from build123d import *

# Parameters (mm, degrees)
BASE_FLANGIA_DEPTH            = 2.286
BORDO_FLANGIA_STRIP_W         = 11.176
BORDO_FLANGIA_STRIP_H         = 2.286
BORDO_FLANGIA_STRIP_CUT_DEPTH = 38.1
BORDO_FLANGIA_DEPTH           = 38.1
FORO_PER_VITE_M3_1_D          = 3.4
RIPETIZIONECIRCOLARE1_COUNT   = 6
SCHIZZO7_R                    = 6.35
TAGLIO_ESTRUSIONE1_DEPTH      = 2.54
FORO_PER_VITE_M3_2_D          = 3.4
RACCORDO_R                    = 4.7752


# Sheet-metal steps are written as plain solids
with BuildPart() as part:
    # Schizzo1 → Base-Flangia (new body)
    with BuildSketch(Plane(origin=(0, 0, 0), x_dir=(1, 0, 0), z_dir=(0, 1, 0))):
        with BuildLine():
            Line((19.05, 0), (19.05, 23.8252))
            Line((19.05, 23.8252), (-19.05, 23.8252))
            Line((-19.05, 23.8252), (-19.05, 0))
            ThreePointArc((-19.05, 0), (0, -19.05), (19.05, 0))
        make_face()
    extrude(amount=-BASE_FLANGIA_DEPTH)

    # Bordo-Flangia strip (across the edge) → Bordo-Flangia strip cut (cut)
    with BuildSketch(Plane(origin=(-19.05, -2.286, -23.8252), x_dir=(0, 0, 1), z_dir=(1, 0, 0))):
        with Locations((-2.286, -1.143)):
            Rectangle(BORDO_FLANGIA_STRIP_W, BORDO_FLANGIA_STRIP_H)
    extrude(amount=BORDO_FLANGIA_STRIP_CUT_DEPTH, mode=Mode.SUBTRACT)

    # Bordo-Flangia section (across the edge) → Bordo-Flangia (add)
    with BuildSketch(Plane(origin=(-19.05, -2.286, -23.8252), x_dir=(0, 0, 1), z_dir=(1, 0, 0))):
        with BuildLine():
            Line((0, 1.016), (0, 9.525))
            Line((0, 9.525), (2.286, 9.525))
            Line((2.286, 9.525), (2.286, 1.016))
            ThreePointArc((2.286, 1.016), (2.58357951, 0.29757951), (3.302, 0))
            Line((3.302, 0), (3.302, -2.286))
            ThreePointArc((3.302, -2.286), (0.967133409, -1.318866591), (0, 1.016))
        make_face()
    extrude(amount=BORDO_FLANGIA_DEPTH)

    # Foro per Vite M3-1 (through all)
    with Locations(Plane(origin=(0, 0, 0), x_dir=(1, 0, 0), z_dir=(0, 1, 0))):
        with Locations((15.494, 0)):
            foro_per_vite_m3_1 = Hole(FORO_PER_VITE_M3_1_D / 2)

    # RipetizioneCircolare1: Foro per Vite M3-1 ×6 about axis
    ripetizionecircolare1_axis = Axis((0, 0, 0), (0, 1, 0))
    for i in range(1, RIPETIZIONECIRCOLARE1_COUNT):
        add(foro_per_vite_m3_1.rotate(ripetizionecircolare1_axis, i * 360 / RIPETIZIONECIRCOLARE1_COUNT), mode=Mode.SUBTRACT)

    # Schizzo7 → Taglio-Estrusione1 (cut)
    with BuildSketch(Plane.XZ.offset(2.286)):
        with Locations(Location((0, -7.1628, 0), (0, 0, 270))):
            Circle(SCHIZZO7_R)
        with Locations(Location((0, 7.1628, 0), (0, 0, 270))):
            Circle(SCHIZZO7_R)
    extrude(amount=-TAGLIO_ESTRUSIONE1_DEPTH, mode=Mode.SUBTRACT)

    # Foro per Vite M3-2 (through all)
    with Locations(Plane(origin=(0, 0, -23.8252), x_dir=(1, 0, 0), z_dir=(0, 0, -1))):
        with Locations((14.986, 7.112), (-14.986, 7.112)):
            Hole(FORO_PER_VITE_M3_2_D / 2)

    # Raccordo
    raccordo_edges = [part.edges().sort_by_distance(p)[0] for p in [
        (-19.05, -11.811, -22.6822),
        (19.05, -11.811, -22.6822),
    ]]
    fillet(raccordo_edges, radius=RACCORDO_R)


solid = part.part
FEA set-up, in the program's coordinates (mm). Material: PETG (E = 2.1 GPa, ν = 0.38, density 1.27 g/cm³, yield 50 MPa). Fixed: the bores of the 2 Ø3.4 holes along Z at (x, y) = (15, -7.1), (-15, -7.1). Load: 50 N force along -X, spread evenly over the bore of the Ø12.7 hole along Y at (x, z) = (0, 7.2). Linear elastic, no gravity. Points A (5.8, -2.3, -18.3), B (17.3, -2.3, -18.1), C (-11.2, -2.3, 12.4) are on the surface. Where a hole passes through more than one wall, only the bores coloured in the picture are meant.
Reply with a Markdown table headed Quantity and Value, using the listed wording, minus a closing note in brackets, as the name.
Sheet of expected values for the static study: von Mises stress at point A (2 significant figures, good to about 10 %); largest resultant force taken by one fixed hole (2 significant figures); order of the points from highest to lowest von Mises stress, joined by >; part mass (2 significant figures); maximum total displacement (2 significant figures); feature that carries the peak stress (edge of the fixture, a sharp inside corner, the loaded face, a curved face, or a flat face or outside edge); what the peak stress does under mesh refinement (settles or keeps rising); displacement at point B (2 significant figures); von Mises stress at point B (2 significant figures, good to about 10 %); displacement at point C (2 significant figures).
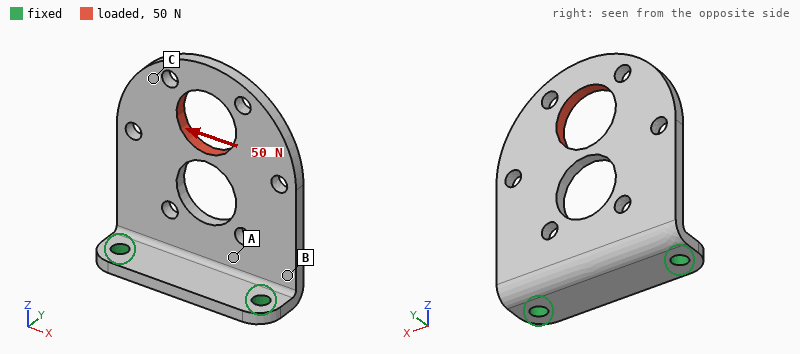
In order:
| Quantity | Value |
|---|---|
| von Mises stress at point A | 4.0 MPa |
| largest resultant force taken by one fixed hole | 56 N |
| order of the points from highest to lowest von Mises stress, joined by > | B > A > C |
| part mass | 4.3 g |
| maximum total displacement | 0.40 mm |
| feature that carries the peak stress | edge of the fixture |
| what the peak stress does under mesh refinement | keeps rising |
| displacement at point B | 0.13 mm |
| von Mises stress at point B | 7.0 MPa |
| displacement at point C | 0.38 mm |
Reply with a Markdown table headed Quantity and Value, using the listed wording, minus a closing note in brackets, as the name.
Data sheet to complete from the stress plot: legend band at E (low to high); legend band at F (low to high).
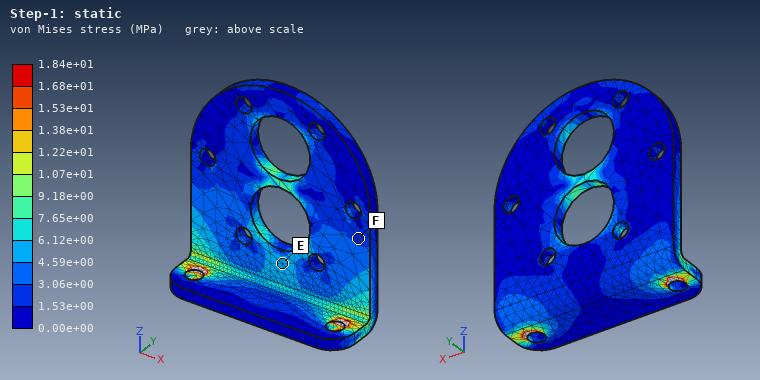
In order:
| Quantity | Value |
|---|---|
| legend band at E | 4.59e+00 to 6.12e+00 MPa |
| legend band at F | 1.53e+00 to 3.06e+00 MPa |
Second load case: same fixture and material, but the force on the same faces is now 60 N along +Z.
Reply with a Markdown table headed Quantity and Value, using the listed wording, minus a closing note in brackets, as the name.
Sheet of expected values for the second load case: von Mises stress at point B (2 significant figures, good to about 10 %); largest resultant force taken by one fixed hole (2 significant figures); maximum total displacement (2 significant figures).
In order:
| Quantity | Value |
|---|---|
| von Mises stress at point B | 2.2 MPa |
| largest resultant force taken by one fixed hole | 30 N |
| maximum total displacement | 0.61 mm |
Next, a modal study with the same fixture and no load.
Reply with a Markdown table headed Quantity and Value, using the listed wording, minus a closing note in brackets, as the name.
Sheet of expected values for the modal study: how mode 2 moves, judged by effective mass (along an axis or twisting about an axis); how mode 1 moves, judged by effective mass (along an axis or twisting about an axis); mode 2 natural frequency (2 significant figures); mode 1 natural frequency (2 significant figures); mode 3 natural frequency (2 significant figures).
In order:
| Quantity | Value |
|---|---|
| how mode 2 moves, judged by effective mass | twisting about Z |
| how mode 1 moves, judged by effective mass | along Y |
| mode 2 natural frequency | 740 Hz |
| mode 1 natural frequency | 280 Hz |
| mode 3 natural frequency | 1400 Hz |
